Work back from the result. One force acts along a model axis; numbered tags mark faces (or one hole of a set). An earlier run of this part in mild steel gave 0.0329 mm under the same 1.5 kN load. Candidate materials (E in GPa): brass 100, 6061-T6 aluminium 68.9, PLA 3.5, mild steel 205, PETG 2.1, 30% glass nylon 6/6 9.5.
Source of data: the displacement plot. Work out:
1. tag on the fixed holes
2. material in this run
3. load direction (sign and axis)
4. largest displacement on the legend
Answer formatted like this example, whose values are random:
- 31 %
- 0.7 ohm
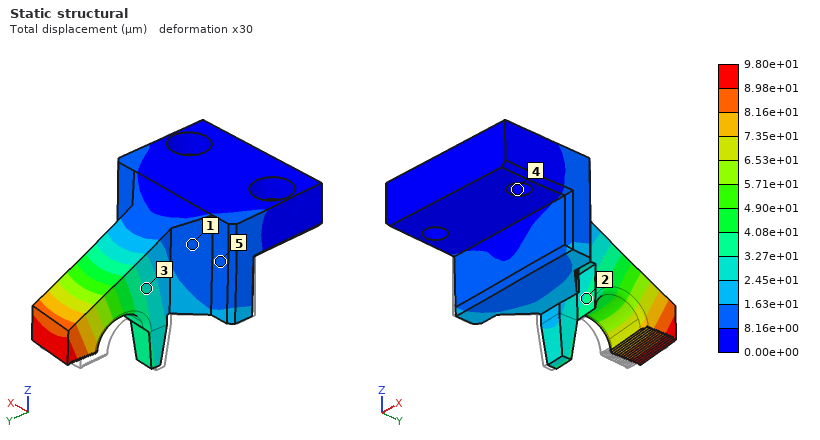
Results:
- 4
- 6061-T6 aluminium
- +X
- 9.80e+01 µm
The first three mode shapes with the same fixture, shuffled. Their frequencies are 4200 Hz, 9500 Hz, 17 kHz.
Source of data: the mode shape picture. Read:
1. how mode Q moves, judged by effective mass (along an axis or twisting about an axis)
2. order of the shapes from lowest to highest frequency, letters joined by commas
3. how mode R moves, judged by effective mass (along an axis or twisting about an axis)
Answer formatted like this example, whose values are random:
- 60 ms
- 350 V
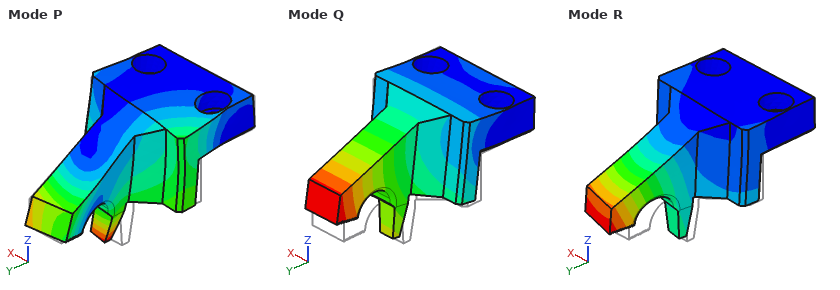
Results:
- along Z
- Q, R, P
- along X
